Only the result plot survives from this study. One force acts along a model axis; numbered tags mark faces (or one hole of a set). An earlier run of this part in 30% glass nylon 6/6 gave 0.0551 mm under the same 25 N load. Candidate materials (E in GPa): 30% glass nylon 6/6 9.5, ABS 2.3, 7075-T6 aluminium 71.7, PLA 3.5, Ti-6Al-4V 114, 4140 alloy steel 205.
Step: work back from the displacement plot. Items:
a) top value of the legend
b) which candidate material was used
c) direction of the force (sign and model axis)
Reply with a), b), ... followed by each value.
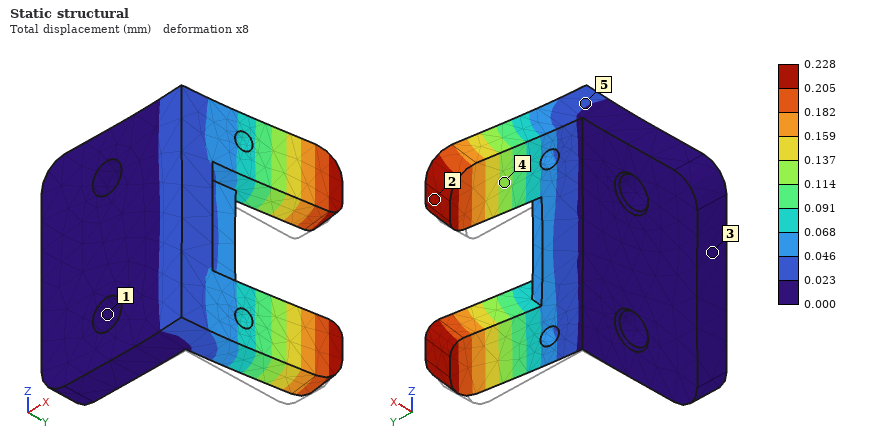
a) 0.228 mm
b) ABS
c) +X
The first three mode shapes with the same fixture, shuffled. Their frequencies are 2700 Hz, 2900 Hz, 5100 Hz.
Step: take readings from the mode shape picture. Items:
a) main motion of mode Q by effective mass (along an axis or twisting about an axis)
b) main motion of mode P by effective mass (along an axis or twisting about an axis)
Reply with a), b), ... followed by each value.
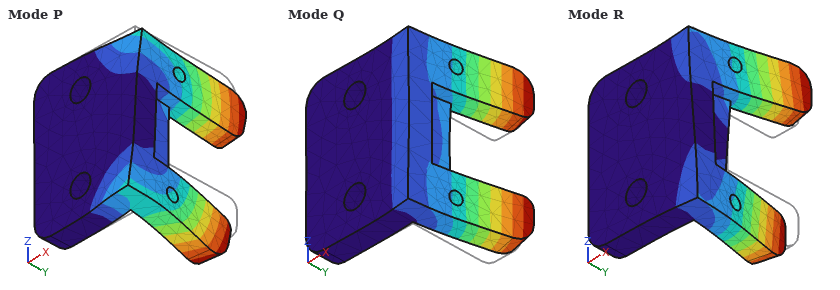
a) along X
b) along Z
